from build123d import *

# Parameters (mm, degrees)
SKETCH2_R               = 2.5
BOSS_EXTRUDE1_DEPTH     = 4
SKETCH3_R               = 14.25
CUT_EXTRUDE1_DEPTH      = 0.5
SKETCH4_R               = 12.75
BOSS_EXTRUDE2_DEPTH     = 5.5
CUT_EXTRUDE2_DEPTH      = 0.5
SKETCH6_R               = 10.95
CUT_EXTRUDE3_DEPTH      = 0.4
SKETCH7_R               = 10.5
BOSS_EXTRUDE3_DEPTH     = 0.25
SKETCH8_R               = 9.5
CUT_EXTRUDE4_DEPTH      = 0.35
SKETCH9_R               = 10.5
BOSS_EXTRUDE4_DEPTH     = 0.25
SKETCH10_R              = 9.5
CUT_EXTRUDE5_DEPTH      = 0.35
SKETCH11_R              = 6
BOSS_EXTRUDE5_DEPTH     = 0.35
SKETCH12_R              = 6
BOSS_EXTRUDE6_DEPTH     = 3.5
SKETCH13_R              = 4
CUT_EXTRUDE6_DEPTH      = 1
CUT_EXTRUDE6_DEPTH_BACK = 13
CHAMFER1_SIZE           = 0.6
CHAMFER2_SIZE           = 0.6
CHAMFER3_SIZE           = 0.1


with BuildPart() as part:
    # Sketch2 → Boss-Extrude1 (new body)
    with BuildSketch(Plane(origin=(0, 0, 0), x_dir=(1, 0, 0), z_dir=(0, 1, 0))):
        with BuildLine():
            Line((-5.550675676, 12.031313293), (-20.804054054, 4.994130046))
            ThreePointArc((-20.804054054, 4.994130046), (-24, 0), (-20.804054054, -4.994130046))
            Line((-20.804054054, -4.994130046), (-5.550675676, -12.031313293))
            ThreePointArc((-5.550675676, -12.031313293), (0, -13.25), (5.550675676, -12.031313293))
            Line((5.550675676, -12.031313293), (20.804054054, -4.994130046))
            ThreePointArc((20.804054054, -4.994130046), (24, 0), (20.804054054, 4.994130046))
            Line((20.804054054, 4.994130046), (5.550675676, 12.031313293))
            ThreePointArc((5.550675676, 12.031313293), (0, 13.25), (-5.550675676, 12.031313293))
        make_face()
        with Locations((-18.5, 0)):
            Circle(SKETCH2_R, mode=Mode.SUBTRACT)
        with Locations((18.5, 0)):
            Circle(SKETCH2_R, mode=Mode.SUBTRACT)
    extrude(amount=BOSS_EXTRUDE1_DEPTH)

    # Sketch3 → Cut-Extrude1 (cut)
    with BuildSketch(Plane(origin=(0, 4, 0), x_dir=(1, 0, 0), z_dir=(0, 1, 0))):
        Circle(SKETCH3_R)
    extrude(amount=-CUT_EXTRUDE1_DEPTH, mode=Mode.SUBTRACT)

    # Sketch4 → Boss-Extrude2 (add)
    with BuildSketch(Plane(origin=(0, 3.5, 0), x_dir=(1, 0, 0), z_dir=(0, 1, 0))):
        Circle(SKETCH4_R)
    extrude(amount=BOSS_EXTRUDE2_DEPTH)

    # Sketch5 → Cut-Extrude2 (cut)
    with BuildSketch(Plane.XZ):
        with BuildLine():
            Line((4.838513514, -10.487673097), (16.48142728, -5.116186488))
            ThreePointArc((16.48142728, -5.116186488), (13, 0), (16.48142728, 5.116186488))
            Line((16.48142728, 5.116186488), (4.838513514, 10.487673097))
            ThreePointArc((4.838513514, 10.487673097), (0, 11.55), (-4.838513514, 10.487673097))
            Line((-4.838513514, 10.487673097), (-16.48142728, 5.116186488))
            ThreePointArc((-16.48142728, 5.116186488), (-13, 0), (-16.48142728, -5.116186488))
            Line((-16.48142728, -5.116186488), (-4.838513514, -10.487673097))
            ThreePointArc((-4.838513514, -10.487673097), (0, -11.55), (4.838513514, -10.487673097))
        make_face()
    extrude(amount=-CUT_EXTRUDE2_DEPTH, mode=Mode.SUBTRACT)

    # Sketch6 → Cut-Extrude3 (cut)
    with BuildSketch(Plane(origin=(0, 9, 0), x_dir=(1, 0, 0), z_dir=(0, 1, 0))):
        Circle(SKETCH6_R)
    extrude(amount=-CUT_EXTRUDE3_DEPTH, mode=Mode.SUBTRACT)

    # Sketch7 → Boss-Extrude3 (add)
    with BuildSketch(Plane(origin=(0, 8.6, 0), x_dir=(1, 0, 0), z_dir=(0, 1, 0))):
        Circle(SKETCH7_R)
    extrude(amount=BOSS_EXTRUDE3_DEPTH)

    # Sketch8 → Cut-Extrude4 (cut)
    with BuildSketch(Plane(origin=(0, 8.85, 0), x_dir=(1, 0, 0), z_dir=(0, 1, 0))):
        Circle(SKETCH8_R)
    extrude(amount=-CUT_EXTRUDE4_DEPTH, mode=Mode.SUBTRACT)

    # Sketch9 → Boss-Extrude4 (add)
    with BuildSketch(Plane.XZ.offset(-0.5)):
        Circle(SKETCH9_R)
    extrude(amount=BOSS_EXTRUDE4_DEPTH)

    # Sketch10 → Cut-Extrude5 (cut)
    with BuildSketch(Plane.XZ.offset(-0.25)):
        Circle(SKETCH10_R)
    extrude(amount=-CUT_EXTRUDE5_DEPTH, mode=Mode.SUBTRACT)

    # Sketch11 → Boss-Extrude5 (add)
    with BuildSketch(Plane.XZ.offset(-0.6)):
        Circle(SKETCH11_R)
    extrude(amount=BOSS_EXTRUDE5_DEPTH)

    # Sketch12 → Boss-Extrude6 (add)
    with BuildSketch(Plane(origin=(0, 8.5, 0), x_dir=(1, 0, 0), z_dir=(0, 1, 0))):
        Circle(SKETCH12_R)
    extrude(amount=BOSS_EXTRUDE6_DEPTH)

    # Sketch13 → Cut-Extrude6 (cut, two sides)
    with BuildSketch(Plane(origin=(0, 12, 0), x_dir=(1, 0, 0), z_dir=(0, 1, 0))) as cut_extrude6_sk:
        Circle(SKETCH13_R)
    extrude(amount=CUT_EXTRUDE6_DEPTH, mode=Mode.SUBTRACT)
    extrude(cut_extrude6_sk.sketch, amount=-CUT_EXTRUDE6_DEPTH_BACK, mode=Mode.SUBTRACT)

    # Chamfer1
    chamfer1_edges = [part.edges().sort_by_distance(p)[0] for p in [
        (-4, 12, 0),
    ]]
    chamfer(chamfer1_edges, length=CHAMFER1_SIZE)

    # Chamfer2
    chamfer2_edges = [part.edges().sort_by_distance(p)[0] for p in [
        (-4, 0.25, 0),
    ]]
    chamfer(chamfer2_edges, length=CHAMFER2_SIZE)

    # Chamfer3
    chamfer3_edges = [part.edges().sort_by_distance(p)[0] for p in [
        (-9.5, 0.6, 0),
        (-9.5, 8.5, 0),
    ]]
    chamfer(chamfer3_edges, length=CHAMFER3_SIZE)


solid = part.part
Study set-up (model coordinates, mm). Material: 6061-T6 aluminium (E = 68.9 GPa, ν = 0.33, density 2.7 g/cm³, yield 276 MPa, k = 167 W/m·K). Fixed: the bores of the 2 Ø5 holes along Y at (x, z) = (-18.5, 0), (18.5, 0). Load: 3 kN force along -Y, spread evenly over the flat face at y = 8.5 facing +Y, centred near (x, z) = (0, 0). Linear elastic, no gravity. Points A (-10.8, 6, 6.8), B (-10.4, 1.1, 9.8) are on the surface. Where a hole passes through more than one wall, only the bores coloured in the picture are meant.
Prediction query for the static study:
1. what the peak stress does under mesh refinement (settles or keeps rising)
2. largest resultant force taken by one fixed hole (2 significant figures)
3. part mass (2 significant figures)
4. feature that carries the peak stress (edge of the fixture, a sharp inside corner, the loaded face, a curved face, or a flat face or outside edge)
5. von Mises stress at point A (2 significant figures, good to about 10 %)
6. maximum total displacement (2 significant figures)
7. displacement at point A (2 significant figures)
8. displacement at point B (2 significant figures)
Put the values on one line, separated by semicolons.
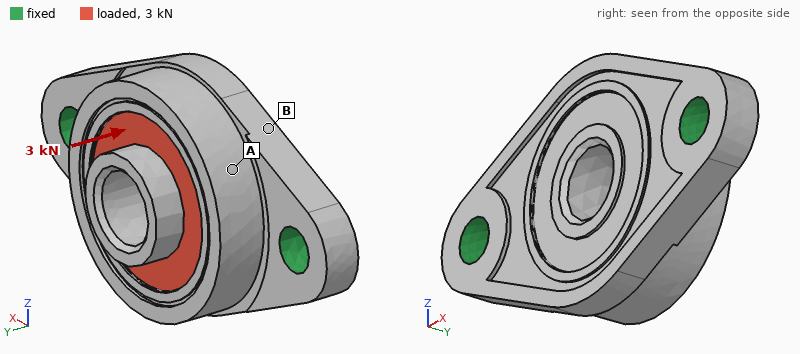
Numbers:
keeps rising; 1.9 kN; 14 g; edge of the fixture; 41 MPa; 37 µm; 23 µm; 25 µm
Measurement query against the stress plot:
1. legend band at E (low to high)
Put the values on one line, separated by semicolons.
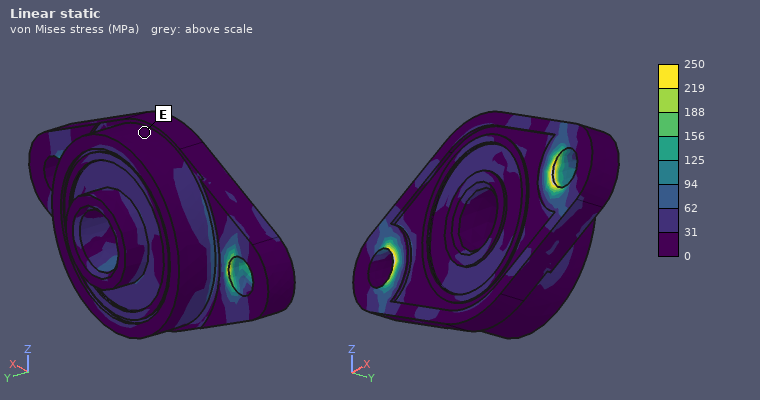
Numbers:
0 to 31 MPa
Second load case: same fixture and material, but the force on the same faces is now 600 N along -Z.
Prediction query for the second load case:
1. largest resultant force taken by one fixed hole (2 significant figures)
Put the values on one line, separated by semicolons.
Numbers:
300 N
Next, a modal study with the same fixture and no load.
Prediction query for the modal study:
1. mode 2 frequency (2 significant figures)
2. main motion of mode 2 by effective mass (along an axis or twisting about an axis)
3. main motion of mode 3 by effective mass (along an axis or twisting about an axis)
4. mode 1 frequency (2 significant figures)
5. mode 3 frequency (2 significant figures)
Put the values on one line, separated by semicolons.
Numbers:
15 kHz; along Y; along Z; 9200 Hz; 25 kHz
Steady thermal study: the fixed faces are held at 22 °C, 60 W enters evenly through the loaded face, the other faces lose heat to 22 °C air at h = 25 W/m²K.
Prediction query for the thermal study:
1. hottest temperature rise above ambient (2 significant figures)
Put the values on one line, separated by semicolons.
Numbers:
35 K
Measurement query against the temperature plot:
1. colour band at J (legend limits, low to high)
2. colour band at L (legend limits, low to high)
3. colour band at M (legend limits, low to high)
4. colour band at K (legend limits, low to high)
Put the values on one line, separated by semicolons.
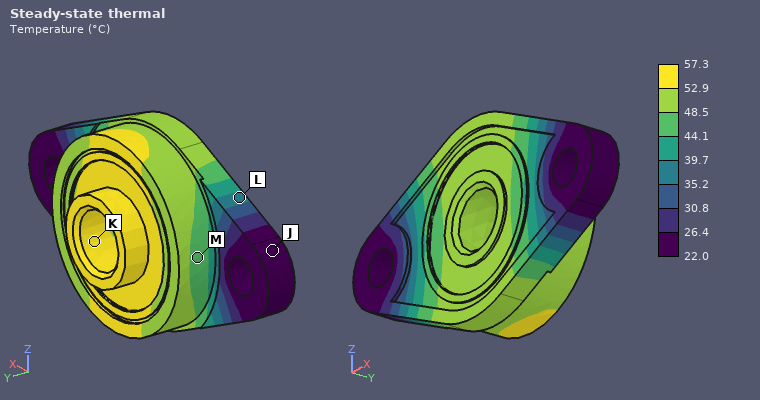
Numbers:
22.0 to 26.4 °C; 35.2 to 39.7 °C; 44.1 to 48.5 °C; 52.9 to 57.3 °C
